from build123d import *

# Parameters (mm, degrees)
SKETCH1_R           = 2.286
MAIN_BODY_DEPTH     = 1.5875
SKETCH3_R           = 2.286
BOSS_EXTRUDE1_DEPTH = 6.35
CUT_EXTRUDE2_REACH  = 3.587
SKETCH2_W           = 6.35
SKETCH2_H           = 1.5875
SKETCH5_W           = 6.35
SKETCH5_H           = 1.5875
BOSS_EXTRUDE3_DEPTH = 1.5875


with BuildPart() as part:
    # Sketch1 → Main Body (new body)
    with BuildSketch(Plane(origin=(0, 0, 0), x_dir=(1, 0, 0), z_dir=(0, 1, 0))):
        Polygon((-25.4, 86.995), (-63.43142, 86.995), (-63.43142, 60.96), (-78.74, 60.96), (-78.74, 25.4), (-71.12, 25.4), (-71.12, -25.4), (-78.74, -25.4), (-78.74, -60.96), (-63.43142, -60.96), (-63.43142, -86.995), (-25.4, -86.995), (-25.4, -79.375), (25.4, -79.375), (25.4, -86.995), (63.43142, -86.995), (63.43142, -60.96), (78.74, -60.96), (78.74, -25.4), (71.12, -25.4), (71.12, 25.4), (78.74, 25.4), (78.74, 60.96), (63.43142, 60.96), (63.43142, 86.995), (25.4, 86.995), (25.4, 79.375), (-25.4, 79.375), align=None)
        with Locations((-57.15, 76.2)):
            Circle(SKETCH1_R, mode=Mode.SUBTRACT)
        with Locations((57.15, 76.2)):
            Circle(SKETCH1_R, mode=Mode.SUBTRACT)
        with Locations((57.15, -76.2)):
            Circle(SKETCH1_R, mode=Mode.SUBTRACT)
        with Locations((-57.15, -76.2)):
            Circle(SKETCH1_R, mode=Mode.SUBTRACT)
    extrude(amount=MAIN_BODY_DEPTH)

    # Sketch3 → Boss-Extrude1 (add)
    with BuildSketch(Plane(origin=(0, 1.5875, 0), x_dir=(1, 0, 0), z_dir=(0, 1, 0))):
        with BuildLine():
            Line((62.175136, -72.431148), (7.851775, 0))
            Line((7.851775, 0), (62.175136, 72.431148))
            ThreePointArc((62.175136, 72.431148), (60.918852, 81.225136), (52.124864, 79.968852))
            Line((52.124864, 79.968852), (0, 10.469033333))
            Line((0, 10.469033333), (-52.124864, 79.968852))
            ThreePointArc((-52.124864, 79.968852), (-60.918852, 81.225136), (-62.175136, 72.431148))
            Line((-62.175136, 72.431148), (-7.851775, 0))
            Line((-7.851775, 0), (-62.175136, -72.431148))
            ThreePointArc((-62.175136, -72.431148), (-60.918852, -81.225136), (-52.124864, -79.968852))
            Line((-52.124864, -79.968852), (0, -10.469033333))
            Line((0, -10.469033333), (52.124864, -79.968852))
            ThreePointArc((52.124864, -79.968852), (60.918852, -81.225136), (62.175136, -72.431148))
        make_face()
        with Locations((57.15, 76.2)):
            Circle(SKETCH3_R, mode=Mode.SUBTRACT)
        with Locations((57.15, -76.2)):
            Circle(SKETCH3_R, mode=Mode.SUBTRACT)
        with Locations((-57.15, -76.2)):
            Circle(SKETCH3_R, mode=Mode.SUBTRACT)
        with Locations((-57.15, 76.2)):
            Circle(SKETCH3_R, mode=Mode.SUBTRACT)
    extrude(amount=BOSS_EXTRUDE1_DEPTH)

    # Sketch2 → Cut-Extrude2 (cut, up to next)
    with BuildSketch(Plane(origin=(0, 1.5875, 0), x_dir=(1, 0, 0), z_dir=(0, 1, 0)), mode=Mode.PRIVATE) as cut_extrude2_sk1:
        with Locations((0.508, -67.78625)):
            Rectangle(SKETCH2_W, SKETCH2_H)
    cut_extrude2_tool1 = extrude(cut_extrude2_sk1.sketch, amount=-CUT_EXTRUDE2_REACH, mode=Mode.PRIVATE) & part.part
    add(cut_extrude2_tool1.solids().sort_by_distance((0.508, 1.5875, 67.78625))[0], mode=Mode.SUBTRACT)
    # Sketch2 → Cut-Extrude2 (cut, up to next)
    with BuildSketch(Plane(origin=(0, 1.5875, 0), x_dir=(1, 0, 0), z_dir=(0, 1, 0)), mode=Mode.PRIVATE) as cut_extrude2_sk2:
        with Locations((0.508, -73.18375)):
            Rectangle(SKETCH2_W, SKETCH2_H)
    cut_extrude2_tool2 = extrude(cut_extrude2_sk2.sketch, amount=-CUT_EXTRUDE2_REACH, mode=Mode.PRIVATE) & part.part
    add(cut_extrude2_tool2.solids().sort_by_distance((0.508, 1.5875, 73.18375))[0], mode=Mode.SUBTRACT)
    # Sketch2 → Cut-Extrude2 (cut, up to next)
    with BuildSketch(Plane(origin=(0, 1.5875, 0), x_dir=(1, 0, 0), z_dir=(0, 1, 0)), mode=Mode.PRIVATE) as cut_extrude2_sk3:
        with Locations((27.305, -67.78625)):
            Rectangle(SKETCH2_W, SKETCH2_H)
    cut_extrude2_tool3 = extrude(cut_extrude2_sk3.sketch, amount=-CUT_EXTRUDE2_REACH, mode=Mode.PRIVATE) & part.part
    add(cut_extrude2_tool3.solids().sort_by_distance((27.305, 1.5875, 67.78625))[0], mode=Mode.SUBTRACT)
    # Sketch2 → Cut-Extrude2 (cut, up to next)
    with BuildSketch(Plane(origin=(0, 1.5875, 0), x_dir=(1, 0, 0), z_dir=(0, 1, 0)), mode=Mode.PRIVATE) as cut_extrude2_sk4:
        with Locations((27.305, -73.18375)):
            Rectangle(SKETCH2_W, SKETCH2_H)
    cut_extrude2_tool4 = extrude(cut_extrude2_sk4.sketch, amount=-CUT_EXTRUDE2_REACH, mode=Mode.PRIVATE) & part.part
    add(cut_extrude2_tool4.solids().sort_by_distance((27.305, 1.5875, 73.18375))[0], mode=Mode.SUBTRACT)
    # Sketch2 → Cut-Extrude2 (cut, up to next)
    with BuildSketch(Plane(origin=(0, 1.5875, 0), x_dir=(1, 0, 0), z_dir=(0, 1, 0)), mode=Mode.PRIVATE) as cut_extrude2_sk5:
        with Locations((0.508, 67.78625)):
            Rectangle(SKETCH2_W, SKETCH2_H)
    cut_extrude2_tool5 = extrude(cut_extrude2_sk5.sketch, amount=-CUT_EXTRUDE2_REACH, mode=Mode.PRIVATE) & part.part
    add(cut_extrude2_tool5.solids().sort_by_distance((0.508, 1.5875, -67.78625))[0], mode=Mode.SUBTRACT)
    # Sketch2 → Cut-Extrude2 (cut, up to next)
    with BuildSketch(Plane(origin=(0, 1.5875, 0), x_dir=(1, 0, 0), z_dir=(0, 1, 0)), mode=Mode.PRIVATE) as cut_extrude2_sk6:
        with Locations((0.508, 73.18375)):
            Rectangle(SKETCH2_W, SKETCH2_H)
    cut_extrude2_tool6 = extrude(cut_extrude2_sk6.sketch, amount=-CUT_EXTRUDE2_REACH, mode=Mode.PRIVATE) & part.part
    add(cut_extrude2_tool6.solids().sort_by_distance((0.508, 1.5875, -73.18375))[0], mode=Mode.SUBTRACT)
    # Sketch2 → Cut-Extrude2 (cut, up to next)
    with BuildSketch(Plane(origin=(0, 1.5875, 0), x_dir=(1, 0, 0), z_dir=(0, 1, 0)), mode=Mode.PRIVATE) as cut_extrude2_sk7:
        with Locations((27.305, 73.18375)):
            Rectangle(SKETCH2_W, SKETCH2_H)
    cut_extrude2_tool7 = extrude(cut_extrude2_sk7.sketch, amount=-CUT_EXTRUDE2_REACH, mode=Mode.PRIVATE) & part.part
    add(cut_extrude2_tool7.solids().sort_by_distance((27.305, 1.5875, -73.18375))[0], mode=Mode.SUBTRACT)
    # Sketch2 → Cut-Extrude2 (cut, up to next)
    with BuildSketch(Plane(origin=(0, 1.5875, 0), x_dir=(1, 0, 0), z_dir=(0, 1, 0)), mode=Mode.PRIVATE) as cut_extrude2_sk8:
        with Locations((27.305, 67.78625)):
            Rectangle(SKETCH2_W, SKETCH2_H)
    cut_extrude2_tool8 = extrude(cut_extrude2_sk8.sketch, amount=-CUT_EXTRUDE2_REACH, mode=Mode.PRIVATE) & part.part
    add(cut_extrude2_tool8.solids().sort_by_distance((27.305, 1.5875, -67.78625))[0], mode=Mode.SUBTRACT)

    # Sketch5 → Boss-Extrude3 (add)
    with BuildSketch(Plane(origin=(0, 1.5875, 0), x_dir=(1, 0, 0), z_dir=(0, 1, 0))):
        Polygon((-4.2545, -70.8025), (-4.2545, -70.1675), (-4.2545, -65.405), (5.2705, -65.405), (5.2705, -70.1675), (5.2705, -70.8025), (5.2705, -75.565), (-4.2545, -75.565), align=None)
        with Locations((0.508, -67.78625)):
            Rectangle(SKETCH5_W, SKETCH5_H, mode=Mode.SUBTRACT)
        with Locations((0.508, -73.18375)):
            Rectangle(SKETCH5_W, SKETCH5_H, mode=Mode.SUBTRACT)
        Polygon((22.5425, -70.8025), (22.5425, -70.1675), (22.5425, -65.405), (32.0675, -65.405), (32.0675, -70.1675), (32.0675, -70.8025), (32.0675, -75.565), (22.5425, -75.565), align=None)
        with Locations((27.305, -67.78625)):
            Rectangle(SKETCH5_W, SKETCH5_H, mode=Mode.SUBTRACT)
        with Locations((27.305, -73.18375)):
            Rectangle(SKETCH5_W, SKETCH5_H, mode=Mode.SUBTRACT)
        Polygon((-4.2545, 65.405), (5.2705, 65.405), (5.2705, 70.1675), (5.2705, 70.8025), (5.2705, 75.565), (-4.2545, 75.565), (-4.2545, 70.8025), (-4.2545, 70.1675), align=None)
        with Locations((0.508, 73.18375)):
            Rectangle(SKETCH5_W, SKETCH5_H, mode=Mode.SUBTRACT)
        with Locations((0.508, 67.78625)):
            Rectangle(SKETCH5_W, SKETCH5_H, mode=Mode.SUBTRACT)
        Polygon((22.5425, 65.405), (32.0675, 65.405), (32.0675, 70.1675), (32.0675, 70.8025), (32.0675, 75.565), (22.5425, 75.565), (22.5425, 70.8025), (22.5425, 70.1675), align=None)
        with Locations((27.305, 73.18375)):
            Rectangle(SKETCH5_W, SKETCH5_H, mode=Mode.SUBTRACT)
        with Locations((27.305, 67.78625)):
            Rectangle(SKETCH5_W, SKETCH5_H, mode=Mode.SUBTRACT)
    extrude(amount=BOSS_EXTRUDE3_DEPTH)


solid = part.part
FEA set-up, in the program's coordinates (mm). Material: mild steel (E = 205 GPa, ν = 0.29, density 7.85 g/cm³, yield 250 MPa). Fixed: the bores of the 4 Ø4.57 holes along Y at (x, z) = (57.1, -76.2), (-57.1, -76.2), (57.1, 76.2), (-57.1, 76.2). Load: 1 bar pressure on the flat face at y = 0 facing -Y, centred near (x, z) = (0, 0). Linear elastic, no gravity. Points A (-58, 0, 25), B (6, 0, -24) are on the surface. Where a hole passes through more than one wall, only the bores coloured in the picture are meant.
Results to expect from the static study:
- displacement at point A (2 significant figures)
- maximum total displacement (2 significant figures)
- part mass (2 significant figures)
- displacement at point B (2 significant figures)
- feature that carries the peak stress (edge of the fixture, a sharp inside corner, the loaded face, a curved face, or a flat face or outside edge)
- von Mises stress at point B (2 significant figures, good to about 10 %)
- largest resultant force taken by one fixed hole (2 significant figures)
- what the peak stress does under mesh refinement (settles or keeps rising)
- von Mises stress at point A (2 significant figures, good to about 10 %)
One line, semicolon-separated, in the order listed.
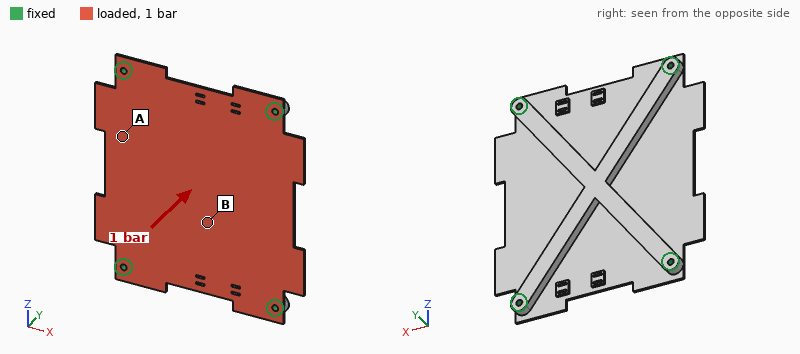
0.26 mm; 0.50 mm; 540 g; 0.085 mm; edge of the fixture; 16 MPa; 990 N; keeps rising; 39 MPa
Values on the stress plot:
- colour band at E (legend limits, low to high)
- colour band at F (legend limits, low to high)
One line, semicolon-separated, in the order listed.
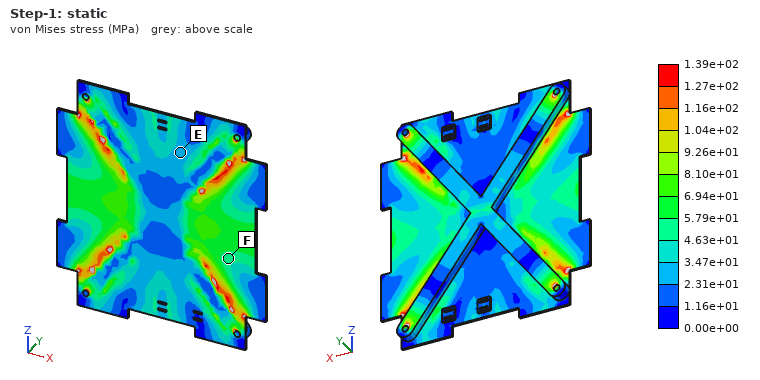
2.31e+01 to 3.47e+01 MPa; 4.63e+01 to 5.79e+01 MPa
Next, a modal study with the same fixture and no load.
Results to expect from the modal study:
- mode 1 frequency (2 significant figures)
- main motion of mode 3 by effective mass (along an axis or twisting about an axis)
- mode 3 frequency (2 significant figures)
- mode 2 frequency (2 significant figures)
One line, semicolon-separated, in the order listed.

870 Hz; along Y; 1300 Hz; 880 Hz
